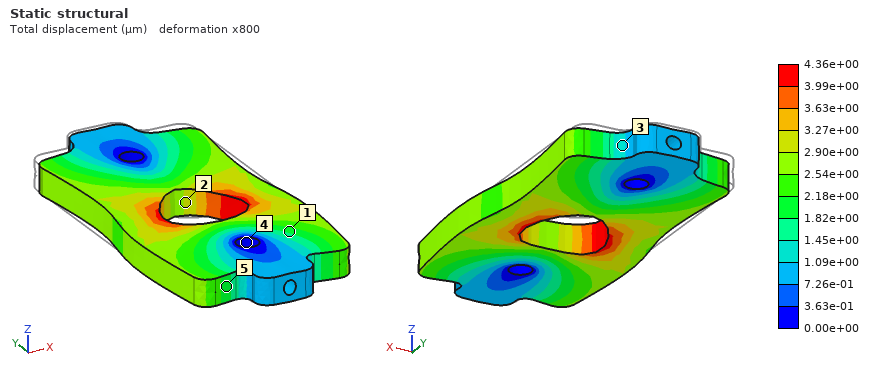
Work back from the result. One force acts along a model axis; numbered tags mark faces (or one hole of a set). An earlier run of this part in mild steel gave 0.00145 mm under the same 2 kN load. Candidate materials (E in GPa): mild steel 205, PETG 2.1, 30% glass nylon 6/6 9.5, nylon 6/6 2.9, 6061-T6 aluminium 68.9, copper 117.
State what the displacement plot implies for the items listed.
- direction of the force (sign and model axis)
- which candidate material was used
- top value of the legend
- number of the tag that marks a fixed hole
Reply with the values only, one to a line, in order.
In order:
-Y
6061-T6 aluminium
4.36e+00 µm
4
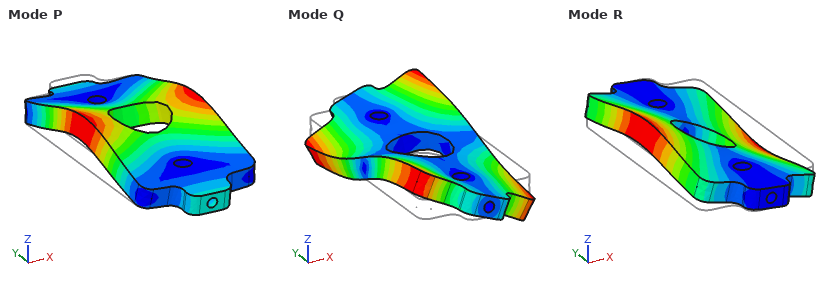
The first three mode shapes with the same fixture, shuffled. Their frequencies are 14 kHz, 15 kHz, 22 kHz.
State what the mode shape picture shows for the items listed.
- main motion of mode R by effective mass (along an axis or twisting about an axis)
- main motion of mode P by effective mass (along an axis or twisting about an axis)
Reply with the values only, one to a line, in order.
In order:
twisting about Y
along Z
